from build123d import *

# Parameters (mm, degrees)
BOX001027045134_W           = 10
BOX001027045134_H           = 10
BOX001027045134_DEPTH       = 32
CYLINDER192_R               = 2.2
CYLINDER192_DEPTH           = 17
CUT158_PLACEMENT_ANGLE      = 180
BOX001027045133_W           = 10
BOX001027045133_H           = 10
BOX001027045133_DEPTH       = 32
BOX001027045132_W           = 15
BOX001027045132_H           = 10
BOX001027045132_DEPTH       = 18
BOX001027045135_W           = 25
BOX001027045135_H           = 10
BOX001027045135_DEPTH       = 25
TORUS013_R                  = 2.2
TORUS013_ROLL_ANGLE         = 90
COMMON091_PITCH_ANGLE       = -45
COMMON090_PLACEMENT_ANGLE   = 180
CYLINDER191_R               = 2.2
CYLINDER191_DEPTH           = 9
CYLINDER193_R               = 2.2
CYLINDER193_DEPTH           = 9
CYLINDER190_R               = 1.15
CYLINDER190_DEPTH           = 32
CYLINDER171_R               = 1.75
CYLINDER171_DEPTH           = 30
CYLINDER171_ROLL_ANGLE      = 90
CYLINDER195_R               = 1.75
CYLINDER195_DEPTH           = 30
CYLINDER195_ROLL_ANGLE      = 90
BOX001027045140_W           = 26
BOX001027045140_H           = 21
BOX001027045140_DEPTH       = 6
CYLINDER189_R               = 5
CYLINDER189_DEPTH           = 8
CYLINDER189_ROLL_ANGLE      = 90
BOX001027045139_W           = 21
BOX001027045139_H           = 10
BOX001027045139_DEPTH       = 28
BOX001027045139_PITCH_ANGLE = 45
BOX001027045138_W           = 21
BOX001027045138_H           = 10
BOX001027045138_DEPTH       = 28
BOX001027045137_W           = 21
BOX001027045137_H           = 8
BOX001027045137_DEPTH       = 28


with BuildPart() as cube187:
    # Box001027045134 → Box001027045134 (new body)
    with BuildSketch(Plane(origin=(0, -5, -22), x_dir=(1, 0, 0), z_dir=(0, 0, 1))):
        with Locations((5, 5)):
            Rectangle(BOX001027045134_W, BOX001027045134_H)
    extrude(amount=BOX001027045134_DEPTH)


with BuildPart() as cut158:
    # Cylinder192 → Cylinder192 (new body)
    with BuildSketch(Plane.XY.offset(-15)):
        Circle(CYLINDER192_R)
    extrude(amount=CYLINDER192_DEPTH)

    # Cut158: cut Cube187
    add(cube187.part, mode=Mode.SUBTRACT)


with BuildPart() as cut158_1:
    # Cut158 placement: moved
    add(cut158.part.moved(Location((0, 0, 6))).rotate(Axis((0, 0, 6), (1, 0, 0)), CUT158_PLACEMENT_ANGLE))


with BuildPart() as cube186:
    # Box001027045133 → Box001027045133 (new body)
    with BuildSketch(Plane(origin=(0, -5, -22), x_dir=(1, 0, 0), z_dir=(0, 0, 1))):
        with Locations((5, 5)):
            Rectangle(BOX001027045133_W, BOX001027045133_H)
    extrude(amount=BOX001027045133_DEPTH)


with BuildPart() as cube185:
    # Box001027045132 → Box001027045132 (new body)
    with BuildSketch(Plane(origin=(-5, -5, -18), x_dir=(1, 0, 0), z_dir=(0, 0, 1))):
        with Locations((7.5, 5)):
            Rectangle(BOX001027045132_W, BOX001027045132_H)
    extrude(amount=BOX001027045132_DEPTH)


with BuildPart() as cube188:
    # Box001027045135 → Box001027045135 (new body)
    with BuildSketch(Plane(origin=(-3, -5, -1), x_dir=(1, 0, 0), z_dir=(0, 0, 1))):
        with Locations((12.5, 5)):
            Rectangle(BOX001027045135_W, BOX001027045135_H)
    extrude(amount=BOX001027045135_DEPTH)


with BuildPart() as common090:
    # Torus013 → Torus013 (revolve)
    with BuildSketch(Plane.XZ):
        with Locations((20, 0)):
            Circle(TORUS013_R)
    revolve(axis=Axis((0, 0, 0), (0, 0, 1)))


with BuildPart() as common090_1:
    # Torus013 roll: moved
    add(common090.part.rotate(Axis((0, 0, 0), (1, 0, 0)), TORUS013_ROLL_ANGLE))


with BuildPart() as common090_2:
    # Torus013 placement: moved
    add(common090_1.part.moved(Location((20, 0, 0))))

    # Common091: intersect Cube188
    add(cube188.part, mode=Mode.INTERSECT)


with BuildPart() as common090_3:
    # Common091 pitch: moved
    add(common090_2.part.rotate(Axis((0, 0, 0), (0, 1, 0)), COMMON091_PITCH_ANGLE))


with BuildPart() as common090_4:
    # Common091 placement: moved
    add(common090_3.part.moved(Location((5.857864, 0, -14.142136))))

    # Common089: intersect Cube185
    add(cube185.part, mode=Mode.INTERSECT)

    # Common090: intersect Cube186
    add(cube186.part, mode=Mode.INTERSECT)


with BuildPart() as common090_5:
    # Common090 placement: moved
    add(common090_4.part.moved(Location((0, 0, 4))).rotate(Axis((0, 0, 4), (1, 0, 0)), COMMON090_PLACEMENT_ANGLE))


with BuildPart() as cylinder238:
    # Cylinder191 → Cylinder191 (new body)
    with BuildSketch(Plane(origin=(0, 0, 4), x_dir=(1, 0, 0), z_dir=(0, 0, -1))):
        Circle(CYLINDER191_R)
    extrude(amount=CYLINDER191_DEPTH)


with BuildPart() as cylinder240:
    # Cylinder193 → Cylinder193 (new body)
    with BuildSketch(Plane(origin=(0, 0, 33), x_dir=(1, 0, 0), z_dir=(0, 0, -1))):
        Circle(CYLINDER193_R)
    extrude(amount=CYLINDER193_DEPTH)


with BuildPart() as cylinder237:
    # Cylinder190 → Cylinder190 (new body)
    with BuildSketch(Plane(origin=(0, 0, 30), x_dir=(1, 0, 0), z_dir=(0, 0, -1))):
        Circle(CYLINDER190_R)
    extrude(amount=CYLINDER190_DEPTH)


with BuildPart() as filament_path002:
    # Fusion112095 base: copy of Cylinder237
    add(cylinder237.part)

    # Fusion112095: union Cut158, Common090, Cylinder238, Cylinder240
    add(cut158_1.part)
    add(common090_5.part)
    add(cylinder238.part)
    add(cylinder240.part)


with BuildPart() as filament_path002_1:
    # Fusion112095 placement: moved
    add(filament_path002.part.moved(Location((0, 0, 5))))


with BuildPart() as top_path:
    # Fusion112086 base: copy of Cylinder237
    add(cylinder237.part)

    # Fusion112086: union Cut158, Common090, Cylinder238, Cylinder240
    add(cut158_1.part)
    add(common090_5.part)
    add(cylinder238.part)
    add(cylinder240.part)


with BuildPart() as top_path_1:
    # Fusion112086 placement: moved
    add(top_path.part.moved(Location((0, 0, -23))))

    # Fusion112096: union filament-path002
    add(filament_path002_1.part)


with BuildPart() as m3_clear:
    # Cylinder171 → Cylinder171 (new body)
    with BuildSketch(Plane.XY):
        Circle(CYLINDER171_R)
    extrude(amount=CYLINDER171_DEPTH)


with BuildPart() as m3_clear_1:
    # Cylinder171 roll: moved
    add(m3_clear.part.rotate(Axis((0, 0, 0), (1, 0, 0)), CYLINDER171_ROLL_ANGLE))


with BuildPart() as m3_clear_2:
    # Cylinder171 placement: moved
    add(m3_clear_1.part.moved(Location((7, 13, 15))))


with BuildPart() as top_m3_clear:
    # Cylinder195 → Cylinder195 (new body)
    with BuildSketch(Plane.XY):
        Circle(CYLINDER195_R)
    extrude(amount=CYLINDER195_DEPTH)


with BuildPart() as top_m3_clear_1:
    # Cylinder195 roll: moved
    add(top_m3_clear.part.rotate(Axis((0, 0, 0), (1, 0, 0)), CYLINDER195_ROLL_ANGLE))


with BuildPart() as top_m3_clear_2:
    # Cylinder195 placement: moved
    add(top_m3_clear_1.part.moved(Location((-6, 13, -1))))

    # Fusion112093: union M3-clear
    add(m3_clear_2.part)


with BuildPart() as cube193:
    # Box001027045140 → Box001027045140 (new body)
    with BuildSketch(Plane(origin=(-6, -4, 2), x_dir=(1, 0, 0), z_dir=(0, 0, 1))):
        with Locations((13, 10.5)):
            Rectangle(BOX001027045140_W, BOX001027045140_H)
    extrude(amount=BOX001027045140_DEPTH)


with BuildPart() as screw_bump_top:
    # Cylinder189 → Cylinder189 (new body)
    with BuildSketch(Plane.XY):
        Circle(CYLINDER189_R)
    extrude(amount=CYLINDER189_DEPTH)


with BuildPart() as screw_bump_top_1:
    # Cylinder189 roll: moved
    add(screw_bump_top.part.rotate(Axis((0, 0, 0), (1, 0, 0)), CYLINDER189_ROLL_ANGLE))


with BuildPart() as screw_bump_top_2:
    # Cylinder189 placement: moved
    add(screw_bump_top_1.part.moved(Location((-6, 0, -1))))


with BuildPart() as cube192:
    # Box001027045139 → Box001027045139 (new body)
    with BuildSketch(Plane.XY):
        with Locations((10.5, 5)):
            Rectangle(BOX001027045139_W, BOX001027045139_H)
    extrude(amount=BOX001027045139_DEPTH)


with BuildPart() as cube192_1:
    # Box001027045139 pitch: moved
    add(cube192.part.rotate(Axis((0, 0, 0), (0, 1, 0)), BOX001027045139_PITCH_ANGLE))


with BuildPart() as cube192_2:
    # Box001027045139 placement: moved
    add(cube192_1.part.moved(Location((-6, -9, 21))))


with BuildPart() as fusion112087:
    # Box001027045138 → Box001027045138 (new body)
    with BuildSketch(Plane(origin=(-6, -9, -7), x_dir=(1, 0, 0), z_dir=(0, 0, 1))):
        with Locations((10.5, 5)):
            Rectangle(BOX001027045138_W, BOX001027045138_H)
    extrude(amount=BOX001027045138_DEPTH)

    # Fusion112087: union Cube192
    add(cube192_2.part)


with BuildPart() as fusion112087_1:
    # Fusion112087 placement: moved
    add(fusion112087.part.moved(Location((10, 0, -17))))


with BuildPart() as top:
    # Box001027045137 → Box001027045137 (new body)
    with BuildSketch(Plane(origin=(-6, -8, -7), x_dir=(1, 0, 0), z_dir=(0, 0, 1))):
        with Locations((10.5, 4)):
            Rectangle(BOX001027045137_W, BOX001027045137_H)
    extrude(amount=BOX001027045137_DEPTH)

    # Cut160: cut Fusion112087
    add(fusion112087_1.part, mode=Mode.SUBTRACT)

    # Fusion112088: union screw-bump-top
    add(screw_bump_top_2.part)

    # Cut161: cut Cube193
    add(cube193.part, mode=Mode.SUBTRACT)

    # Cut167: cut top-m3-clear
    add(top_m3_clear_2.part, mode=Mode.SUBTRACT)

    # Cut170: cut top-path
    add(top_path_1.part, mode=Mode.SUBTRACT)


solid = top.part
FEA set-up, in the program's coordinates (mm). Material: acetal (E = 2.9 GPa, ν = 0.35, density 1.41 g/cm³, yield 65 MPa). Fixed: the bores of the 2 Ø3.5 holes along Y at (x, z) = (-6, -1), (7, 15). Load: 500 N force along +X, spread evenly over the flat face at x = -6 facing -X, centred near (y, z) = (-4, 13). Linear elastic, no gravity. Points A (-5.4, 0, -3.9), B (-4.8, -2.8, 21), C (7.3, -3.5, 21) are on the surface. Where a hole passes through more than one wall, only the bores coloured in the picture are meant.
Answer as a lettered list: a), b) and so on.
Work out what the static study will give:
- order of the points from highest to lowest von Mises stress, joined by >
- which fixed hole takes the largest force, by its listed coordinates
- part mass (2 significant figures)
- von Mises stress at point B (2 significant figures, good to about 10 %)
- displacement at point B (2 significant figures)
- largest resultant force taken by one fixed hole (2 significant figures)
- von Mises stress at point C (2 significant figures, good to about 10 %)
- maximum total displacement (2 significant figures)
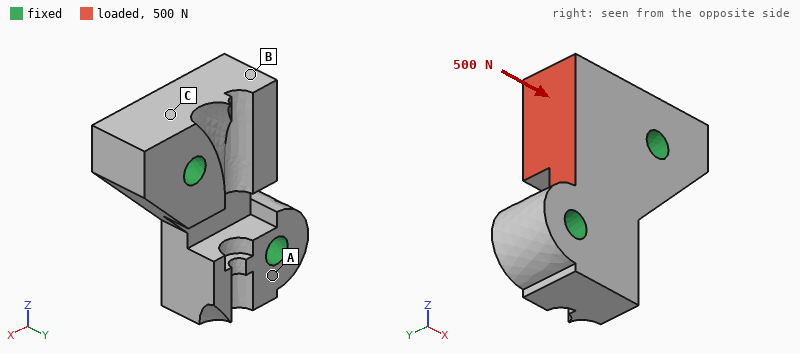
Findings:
a) B > C > A
b) (7, 15)
c) 4.2 g
d) 5.4 MPa
e) 38 µm
f) 430 N
g) 3.2 MPa
h) 55 µm
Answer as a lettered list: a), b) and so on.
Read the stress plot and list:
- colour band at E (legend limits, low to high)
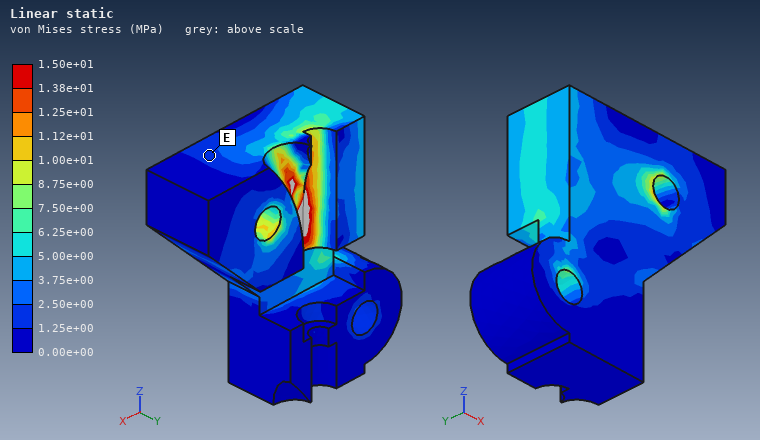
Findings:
a) 1.25e+00 to 2.50e+00 MPa
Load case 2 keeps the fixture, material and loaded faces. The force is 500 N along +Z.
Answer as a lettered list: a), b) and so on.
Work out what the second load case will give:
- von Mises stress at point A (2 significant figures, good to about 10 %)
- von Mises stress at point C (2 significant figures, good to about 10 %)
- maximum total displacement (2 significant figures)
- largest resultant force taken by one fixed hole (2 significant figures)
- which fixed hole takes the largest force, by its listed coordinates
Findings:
a) 3.2 MPa
b) 4.8 MPa
c) 0.14 mm
d) 330 N
e) (-6, -1)
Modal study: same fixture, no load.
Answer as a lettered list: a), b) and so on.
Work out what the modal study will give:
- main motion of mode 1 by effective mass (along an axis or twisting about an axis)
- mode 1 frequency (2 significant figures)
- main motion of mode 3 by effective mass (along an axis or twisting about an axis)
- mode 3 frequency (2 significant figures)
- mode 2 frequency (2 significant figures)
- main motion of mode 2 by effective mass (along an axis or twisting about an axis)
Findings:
a) along Y
b) 8500 Hz
c) along Y
d) 14 kHz
e) 12 kHz
f) along Z
